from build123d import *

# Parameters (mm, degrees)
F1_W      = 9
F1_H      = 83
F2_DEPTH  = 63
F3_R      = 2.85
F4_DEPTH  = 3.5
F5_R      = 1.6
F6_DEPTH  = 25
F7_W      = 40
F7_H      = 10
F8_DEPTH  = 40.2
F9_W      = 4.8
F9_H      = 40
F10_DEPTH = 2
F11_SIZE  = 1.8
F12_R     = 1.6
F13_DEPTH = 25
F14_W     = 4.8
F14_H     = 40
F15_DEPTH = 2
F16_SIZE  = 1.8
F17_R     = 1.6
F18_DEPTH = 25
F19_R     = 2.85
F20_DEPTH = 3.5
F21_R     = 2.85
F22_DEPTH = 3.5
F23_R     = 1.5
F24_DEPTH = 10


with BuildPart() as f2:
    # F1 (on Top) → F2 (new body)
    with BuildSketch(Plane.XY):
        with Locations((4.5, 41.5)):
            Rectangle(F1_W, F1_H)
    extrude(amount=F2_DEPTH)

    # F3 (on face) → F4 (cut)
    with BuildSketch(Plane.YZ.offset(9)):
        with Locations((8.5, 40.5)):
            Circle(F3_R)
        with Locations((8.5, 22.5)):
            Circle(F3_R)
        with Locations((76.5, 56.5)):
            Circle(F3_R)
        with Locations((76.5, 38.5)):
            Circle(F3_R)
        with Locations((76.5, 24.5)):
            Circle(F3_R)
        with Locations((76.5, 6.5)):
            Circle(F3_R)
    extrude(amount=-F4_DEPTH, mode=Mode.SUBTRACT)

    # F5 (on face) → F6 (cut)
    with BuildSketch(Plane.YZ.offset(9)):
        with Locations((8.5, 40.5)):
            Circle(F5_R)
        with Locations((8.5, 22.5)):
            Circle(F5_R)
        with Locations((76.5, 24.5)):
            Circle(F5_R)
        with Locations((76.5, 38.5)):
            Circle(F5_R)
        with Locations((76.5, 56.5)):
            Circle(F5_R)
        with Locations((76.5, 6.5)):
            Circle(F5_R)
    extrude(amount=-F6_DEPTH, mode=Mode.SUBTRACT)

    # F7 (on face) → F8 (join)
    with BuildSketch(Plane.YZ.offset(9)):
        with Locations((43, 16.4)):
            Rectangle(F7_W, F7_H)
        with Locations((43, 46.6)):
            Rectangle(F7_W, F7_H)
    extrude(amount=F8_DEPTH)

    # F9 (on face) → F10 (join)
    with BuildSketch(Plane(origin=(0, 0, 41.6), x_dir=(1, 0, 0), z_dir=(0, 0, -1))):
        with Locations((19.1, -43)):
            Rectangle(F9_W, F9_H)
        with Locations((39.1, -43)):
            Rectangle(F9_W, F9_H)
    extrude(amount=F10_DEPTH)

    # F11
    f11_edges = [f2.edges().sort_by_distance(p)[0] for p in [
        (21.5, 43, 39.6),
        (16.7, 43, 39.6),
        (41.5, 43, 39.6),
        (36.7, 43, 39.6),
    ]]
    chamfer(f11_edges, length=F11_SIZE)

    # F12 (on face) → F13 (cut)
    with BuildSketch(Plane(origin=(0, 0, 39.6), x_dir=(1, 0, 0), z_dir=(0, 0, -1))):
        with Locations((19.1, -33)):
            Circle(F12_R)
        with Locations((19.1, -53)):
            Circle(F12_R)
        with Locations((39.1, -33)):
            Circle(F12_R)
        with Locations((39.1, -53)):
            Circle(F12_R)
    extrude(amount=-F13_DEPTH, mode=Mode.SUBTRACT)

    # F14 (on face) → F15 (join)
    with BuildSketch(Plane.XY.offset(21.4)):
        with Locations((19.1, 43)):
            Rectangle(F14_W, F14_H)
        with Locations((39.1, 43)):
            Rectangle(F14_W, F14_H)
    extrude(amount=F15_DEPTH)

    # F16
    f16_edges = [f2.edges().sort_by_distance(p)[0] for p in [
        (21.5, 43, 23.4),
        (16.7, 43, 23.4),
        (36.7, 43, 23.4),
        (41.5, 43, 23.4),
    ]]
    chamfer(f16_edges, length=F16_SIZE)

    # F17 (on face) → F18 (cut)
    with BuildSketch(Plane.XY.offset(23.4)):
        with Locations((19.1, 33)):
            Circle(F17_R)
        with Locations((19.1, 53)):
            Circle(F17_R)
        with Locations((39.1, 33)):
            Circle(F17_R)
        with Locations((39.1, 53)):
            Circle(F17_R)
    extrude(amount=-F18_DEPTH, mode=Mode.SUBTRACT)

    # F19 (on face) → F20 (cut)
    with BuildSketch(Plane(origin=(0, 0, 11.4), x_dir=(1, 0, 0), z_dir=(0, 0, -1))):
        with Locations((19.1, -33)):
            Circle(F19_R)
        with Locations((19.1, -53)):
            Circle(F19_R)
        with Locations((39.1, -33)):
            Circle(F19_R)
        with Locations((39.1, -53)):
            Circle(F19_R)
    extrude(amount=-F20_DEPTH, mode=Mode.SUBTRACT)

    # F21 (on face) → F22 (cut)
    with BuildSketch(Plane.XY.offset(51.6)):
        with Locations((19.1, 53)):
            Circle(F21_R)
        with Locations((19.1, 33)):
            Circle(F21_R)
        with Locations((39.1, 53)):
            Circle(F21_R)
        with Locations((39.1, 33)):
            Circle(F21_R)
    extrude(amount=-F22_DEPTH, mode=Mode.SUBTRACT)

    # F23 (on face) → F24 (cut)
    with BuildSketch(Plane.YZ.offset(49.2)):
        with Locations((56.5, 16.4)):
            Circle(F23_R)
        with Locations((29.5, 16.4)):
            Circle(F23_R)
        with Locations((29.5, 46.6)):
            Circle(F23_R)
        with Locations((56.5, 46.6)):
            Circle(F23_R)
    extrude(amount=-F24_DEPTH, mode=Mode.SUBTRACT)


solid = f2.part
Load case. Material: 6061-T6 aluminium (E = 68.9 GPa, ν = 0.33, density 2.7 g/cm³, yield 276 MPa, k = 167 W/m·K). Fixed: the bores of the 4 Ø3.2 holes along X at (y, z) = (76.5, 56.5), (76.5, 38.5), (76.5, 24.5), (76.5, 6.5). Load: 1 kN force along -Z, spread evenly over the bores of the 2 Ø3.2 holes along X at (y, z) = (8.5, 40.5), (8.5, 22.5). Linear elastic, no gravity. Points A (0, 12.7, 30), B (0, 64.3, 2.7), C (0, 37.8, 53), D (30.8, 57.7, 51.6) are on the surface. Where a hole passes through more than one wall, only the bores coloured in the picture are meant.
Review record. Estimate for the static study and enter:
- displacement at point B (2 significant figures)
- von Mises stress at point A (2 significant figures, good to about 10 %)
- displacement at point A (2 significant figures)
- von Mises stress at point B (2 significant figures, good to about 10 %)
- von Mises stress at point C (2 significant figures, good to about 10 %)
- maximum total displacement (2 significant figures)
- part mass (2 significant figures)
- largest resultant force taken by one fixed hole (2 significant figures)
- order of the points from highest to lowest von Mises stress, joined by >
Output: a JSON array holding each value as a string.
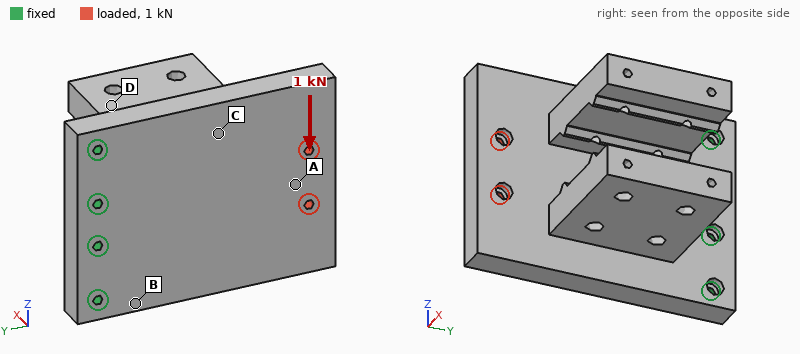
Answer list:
["4.5 µm", "7.0 MPa", "17 µm", "11 MPa", "5.3 MPa", "24 µm", "210 g", "1.3 kN", "B > A > C > D"]
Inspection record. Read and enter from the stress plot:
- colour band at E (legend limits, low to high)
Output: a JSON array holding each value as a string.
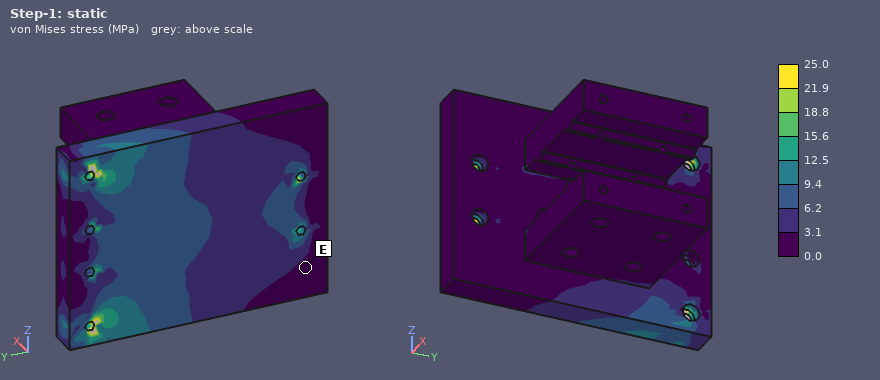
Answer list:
["0.0 to 3.1 MPa"]
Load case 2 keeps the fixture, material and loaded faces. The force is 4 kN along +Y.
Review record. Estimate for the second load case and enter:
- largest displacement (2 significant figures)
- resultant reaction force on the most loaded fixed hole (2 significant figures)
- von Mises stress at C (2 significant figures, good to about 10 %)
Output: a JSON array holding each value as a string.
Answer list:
["56 µm", "1.1 kN", "10 MPa"]
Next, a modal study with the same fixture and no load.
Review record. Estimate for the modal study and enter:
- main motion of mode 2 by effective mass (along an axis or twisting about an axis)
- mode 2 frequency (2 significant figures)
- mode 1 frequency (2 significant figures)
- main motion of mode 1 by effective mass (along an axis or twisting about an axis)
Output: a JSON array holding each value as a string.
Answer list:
["along Z", "2100 Hz", "840 Hz", "along X"]
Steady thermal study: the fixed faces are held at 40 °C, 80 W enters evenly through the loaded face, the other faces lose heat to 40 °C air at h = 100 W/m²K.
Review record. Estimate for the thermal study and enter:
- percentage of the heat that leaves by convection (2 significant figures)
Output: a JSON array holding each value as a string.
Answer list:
["46 %"]
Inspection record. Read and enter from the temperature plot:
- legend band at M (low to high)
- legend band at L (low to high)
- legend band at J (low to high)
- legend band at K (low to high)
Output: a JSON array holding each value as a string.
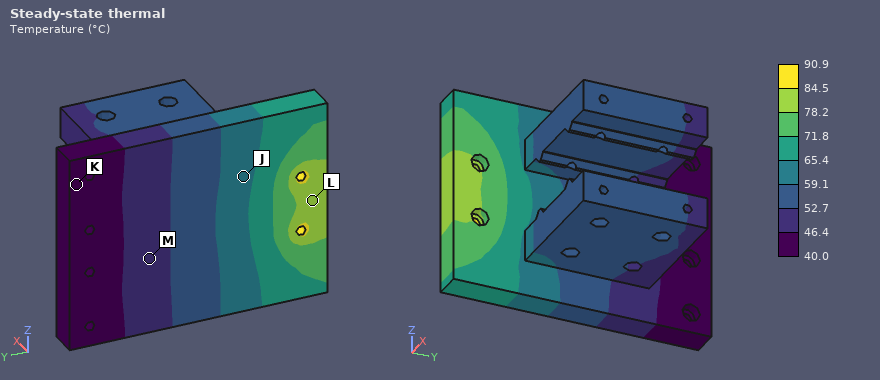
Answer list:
["46.4 to 52.7 °C", "78.2 to 84.5 °C", "59.1 to 65.4 °C", "40.0 to 46.4 °C"]
